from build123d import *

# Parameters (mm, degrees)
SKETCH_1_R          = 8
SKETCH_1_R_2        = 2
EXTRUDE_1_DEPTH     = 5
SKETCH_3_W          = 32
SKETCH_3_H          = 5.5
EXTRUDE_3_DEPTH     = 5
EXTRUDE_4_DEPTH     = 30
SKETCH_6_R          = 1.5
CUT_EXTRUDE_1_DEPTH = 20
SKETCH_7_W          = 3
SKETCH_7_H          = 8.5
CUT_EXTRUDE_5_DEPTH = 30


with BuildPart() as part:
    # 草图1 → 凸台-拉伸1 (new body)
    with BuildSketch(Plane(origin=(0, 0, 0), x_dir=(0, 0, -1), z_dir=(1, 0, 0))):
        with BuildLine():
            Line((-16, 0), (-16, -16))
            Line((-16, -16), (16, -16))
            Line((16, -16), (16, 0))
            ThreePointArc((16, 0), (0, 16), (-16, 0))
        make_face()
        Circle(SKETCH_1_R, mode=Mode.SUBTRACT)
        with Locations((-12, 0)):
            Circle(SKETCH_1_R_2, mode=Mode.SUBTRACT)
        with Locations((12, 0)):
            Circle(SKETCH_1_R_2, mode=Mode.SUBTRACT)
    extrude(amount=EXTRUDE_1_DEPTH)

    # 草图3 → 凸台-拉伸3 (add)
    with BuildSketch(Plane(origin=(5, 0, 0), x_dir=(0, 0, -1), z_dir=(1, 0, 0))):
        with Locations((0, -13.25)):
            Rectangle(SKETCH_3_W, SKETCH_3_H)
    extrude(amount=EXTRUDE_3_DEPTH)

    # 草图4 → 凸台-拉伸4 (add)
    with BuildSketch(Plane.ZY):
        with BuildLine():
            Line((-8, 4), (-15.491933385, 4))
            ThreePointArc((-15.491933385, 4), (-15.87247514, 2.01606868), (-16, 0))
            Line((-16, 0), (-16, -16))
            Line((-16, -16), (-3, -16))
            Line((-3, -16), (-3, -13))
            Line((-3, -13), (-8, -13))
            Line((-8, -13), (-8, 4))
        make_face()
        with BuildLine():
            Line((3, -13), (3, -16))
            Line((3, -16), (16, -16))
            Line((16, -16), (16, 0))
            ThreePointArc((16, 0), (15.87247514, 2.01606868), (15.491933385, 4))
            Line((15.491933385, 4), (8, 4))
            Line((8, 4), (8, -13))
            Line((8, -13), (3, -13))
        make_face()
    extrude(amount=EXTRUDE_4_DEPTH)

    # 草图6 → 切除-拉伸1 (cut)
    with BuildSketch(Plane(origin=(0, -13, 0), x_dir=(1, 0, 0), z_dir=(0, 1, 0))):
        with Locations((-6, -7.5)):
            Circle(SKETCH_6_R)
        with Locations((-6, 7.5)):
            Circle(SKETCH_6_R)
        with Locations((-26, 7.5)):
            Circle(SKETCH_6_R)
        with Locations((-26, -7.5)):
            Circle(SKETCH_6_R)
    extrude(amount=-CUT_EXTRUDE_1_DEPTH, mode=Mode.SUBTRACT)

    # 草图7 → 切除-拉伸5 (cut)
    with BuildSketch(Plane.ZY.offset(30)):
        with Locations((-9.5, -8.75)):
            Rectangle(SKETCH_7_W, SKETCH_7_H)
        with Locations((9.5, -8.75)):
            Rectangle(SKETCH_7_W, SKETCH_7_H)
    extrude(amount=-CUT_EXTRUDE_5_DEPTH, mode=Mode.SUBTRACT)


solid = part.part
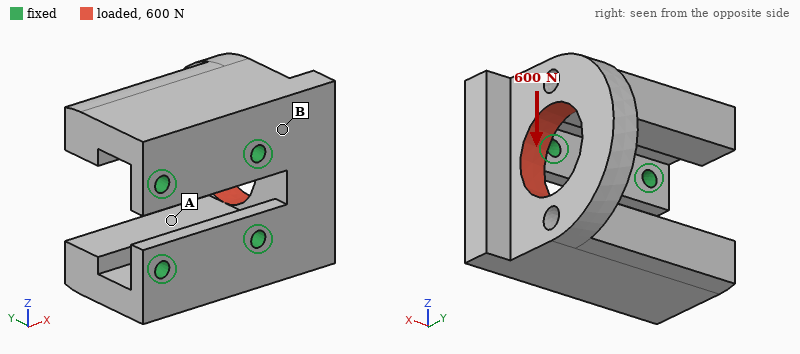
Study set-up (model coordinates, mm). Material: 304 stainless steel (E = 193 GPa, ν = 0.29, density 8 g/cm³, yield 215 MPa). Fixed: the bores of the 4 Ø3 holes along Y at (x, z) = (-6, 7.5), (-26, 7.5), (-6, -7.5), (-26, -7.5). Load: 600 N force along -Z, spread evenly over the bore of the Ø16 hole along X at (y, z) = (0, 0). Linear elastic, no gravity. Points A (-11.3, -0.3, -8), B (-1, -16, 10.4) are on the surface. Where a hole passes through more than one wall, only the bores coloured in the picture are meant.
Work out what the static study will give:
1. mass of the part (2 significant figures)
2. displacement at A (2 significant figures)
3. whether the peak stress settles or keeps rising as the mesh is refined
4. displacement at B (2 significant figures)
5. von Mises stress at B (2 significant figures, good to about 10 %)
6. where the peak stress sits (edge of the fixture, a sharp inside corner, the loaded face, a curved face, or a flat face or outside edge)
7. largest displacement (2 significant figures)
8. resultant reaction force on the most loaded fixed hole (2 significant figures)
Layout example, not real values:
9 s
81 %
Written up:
110 g
6.7 µm
keeps rising
2.3 µm
22 MPa
edge of the fixture
14 µm
540 N
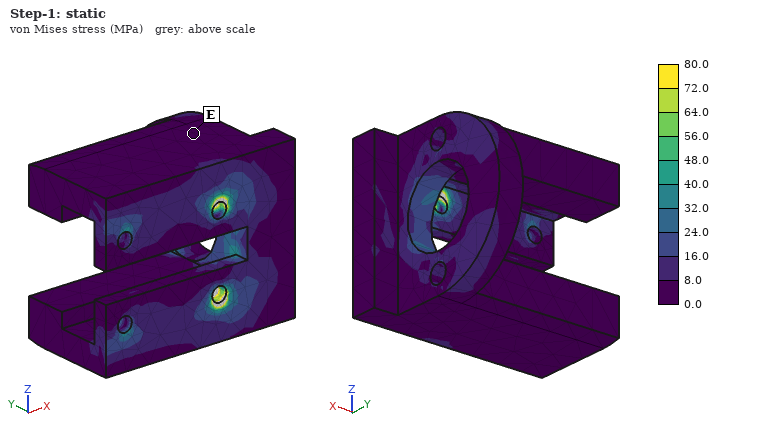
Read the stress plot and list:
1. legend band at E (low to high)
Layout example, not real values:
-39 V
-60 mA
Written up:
0.0 to 8.0 MPa
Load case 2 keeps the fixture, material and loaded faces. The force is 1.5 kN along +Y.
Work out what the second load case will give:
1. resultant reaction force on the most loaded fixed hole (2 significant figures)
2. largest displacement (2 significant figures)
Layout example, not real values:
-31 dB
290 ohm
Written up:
1.0 kN
14 µm
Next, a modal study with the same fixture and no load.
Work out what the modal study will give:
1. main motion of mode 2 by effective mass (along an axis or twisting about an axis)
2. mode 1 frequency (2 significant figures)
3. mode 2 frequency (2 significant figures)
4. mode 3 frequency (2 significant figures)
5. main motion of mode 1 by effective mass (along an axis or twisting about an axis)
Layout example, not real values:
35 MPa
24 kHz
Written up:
along X
5000 Hz
6900 Hz
8800 Hz
along Z
